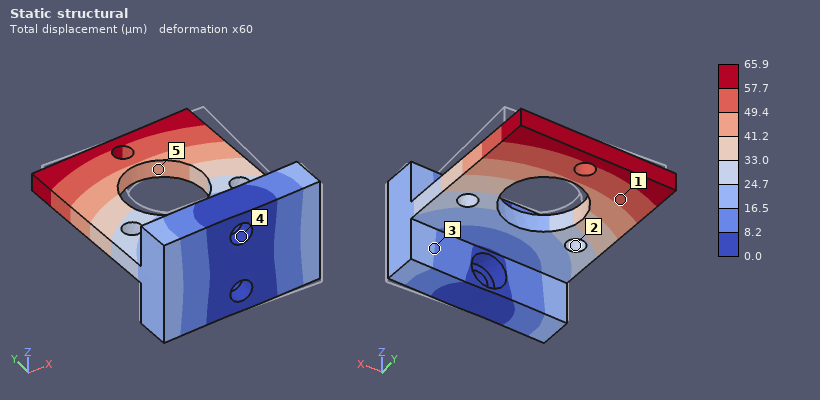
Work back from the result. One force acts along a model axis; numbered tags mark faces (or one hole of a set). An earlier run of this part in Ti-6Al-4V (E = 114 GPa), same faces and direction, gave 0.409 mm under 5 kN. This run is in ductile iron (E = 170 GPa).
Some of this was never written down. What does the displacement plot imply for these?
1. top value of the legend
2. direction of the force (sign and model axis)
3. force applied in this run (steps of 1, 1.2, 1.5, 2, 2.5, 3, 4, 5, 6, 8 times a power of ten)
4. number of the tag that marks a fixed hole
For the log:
65.9 µm
-X
1.2 kN
4
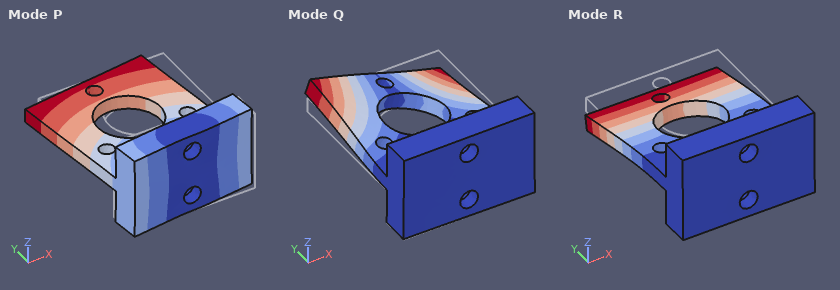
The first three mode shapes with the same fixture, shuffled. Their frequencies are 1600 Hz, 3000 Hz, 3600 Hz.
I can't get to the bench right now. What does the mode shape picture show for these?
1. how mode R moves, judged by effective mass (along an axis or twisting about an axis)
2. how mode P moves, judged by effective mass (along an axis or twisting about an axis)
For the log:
along Z
along X
